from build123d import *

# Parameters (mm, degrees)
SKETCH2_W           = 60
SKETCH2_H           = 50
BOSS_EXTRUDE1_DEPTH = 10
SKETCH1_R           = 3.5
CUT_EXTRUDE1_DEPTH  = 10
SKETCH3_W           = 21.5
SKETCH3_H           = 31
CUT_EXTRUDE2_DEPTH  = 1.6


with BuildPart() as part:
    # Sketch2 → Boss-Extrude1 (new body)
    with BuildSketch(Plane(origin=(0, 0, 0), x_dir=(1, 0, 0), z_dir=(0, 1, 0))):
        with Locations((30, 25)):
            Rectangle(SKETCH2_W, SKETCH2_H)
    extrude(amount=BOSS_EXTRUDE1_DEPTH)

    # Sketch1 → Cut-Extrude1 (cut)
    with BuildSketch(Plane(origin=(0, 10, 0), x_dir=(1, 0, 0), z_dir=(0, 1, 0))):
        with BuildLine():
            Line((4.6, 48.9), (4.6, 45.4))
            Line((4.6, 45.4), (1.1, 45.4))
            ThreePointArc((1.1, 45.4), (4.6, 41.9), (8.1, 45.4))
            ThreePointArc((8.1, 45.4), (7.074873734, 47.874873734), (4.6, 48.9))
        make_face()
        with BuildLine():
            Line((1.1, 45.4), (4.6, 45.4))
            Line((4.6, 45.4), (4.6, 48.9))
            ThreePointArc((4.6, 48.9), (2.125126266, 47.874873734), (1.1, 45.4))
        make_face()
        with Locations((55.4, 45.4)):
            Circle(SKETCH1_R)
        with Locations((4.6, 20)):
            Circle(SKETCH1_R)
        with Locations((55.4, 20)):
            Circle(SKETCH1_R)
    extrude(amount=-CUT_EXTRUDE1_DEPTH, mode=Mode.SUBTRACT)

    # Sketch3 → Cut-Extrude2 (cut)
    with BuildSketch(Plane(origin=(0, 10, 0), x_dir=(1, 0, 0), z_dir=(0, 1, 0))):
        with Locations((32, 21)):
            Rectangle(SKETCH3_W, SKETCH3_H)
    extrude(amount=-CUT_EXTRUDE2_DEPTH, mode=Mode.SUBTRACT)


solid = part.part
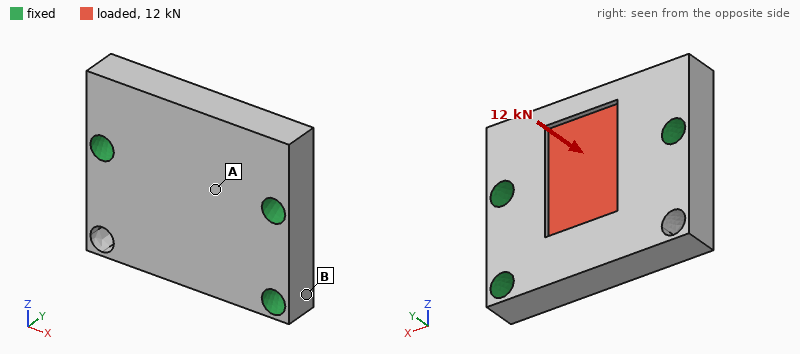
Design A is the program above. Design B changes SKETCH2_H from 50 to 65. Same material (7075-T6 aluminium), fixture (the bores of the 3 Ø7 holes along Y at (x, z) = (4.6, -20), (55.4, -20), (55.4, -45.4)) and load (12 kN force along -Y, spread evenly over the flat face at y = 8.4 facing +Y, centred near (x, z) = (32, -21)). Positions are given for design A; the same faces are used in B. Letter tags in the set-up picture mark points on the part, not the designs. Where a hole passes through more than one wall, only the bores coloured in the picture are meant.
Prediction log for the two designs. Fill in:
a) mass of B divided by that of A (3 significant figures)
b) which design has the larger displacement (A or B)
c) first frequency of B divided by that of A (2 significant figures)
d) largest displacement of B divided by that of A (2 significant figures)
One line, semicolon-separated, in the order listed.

1.33; A; 0.71; 0.90
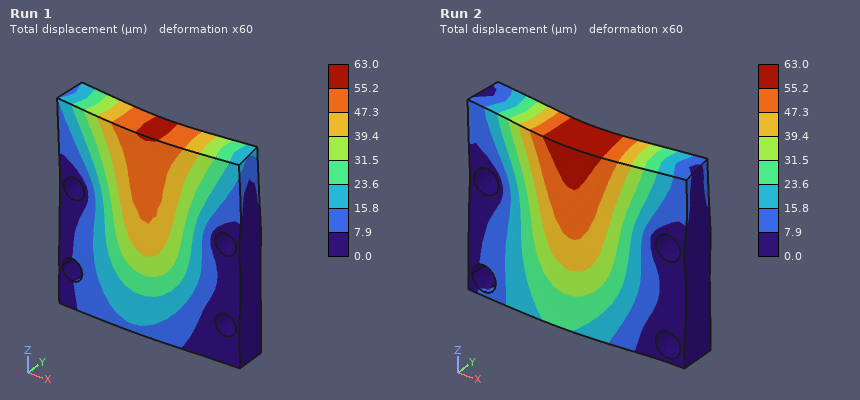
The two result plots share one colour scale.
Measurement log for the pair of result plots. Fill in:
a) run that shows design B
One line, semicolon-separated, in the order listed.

Run 1
